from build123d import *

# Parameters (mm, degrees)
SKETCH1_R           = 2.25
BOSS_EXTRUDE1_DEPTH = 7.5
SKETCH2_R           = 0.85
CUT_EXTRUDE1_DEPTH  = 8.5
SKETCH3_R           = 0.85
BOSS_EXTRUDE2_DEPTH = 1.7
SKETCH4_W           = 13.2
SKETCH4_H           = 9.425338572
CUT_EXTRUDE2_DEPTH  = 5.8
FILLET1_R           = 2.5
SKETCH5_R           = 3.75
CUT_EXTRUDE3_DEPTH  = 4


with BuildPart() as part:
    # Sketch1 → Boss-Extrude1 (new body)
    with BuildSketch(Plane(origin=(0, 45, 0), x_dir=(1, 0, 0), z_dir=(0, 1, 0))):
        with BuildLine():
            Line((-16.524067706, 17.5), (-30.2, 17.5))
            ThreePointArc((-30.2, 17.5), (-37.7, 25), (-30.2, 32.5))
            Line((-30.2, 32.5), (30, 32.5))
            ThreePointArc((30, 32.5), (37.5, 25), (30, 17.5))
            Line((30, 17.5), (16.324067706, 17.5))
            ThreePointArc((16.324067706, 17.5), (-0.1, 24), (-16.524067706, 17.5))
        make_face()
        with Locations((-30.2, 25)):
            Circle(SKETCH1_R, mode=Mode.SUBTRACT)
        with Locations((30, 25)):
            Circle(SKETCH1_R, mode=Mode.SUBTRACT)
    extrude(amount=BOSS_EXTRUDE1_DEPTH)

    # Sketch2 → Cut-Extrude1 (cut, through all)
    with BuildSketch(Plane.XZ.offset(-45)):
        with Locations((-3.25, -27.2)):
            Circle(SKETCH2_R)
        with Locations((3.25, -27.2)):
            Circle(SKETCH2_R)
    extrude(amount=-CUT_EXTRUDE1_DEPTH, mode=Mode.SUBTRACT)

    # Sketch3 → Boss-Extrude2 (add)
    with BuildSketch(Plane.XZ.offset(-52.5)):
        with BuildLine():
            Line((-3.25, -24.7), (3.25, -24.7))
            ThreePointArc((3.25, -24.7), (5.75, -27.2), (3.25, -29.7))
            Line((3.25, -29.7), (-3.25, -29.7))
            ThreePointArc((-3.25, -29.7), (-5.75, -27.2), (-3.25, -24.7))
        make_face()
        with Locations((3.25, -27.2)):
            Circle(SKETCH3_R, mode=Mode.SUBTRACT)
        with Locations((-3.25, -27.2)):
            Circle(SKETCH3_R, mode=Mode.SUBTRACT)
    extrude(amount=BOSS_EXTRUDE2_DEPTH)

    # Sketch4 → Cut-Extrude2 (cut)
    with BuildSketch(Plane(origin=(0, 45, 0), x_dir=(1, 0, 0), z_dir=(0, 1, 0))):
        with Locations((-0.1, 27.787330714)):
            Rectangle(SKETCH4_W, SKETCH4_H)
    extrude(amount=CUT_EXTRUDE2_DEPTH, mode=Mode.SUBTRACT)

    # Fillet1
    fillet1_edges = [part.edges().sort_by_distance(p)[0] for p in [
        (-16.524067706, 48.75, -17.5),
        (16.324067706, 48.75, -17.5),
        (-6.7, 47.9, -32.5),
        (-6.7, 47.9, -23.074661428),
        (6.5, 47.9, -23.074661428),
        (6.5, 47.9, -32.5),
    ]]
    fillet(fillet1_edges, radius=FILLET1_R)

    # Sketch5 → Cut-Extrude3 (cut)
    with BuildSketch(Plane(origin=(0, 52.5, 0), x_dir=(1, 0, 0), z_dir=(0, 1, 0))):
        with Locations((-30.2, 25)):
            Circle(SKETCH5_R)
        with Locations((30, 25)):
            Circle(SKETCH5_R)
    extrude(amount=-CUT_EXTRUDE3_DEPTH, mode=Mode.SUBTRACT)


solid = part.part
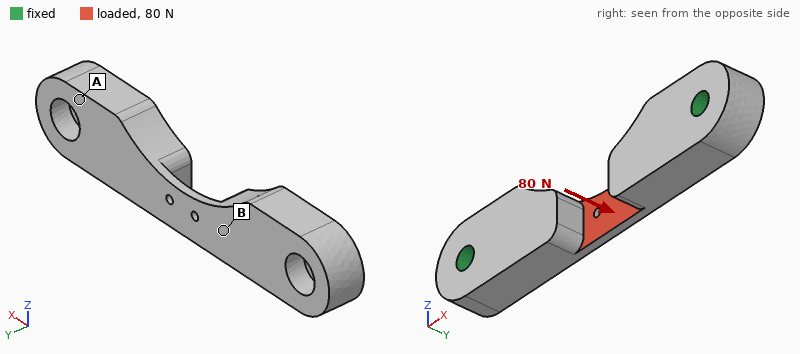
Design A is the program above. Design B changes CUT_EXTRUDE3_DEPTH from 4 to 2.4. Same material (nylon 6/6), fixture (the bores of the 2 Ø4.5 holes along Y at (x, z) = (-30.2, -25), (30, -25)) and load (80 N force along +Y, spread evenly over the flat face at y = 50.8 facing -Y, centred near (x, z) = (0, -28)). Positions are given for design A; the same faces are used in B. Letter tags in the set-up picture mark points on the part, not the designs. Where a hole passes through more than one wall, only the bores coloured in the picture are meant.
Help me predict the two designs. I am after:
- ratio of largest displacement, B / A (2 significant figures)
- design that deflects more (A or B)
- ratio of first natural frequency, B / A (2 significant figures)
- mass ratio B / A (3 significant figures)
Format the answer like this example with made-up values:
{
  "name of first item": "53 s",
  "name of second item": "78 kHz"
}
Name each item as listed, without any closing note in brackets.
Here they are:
{
  "ratio of largest displacement, B / A": "0.89",
  "design that deflects more": "A",
  "ratio of first natural frequency, B / A": "1.2",
  "mass ratio B / A": "1.02"
}
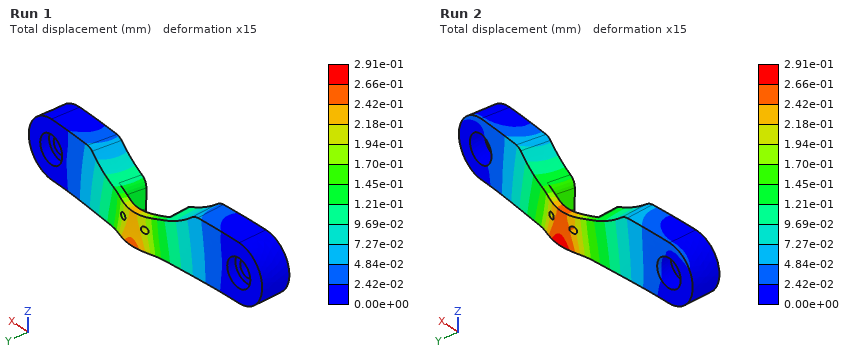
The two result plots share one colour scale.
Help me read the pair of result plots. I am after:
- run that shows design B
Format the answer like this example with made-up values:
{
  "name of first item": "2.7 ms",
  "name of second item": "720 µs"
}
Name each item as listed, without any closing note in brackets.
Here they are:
{
  "run that shows design B": "Run 1"
}
